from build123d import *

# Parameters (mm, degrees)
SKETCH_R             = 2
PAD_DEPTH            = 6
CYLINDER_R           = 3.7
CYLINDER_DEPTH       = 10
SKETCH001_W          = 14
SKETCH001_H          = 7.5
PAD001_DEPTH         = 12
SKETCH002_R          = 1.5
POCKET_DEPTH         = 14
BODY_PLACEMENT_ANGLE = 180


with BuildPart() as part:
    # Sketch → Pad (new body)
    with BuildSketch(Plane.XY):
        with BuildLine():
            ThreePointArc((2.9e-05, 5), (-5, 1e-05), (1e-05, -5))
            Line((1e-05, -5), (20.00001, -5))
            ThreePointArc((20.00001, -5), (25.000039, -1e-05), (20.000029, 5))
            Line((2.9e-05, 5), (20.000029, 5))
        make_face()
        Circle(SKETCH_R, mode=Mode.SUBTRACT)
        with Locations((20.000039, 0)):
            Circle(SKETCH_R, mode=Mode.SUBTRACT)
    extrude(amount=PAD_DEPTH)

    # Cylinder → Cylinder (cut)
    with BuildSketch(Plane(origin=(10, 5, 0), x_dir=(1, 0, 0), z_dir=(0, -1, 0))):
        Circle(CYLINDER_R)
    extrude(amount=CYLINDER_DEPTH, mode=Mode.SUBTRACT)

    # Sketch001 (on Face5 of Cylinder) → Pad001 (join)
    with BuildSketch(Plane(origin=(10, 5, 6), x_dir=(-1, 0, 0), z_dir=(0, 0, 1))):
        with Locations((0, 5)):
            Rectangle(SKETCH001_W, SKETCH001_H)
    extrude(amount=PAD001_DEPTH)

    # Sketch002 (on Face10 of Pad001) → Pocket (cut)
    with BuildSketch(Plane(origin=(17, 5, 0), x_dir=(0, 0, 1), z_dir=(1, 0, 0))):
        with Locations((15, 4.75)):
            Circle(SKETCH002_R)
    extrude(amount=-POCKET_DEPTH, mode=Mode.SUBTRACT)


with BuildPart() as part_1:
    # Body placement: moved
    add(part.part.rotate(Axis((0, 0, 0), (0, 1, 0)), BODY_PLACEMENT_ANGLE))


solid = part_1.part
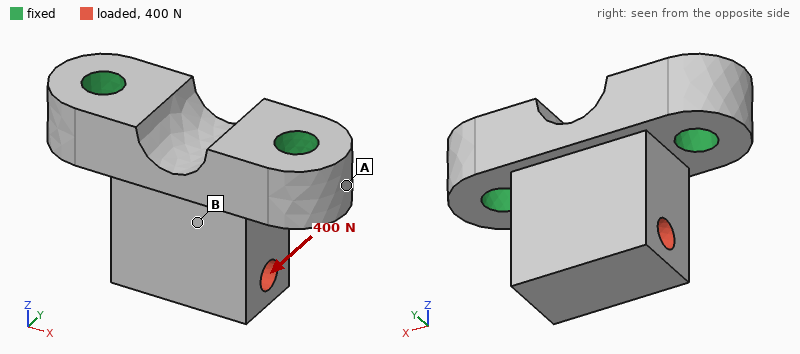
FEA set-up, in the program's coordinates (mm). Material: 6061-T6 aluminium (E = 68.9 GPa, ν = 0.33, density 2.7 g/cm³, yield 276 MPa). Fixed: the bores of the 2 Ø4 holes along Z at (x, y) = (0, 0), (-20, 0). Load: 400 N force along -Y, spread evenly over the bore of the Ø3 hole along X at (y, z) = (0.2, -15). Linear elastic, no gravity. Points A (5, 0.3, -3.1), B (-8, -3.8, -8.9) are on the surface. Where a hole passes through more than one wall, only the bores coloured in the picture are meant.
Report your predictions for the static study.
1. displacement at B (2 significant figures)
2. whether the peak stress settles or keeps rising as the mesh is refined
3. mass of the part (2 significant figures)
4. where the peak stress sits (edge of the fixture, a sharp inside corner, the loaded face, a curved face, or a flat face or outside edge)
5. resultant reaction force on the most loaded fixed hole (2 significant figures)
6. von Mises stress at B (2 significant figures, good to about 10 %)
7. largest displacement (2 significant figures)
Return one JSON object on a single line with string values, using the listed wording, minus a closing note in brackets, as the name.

{"displacement at B": "8.2 µm", "whether the peak stress settles or keeps rising as the mesh is refined": "keeps rising", "mass of the part": "6.7 g", "where the peak stress sits": "edge of the fixture", "resultant reaction force on the most loaded fixed hole": "200 N", "von Mises stress at B": "16 MPa", "largest displacement": "21 µm"}
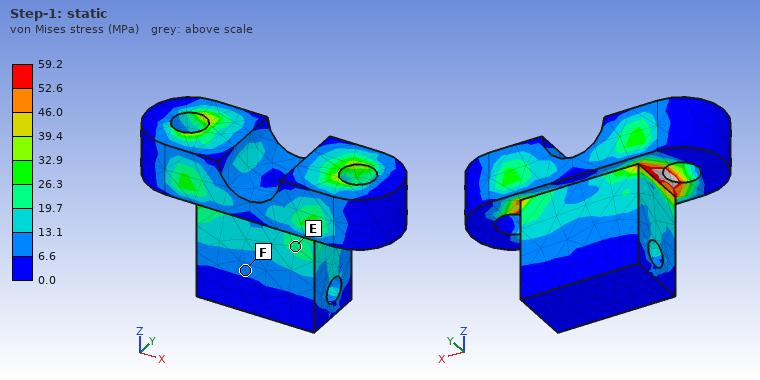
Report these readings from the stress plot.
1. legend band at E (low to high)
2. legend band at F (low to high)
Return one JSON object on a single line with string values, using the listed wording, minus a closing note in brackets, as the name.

{"legend band at E": "19.7 to 26.3 MPa", "legend band at F": "6.6 to 13.1 MPa"}
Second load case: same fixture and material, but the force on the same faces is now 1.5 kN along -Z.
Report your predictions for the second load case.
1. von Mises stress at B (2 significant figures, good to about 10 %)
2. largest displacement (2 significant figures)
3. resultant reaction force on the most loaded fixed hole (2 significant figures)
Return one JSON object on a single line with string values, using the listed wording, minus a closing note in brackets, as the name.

{"von Mises stress at B": "9.6 MPa", "largest displacement": "6.5 µm", "resultant reaction force on the most loaded fixed hole": "840 N"}
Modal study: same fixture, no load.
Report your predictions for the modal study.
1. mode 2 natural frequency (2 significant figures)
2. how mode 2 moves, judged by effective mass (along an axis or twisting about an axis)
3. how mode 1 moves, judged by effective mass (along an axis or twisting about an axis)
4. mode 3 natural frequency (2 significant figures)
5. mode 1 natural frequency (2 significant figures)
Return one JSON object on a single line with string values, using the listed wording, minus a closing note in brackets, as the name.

{"mode 2 natural frequency": "36 kHz", "how mode 2 moves, judged by effective mass": "along X", "how mode 1 moves, judged by effective mass": "along Y", "mode 3 natural frequency": "46 kHz", "mode 1 natural frequency": "18 kHz"}
